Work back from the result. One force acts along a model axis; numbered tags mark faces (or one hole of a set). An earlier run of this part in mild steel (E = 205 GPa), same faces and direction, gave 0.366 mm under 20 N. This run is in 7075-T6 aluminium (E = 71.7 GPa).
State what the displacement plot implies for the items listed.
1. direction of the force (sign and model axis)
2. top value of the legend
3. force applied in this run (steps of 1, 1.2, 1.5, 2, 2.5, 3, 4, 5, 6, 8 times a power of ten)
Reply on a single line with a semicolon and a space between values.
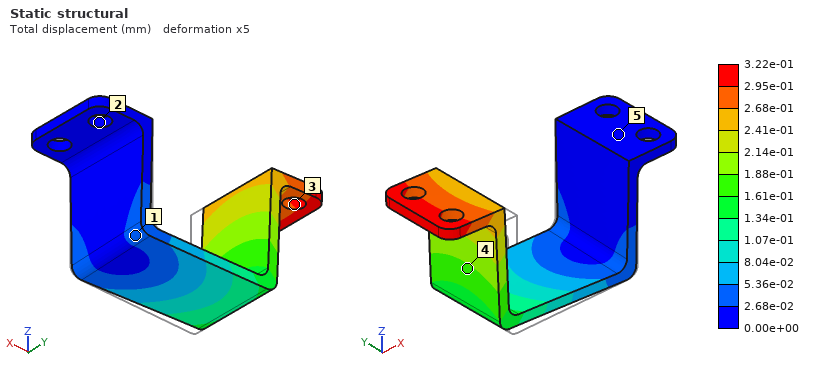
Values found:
+Y; 3.22e-01 mm; 6 N
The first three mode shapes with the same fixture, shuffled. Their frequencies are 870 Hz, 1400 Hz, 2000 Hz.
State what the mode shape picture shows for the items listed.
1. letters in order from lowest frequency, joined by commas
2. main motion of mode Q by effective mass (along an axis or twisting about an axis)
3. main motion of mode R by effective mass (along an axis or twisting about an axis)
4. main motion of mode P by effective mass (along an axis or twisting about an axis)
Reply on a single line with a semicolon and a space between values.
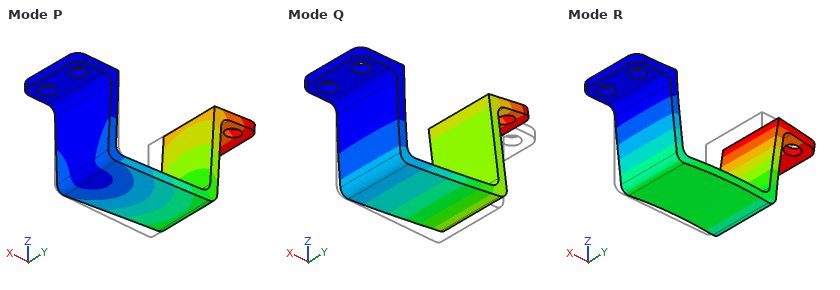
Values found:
Q, P, R; along Z; along X; along Y
